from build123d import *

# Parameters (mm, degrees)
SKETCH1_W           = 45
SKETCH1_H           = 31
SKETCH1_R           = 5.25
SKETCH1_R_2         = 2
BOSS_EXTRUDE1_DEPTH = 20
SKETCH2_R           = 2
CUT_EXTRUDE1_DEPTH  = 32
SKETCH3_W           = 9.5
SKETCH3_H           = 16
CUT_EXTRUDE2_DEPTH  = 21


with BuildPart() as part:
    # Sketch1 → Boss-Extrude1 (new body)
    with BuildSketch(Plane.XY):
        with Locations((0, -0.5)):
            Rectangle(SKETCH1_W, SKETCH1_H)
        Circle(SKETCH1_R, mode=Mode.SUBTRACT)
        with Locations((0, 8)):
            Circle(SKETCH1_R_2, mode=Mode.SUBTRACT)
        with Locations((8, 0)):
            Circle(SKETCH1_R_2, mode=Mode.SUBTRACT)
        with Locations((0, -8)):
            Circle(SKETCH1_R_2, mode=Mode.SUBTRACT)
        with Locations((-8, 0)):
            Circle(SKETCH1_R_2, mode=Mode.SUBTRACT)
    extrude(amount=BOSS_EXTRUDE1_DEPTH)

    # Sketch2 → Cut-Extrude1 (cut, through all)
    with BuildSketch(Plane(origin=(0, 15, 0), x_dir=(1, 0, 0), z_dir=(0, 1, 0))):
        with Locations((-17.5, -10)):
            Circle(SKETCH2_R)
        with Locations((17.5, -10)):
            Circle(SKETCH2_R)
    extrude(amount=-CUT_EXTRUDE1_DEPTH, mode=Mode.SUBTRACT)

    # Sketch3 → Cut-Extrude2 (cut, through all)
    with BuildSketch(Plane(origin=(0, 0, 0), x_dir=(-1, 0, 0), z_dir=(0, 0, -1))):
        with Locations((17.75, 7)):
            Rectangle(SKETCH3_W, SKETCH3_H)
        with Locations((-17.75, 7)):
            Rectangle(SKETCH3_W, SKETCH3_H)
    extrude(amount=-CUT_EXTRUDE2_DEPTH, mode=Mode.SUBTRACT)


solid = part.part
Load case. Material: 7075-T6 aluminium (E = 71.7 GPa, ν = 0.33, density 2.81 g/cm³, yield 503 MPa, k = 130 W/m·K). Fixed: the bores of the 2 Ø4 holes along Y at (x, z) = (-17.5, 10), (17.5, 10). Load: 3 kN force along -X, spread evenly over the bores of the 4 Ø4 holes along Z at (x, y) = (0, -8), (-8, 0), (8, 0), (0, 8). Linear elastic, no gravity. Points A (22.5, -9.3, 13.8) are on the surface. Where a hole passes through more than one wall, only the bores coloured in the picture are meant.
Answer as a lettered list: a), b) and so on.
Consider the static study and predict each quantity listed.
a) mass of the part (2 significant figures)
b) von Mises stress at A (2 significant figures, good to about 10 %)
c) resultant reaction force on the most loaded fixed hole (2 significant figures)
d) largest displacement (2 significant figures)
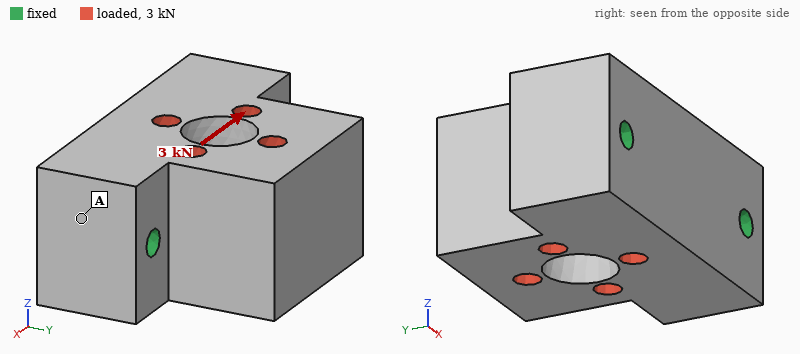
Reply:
a) 53 g
b) 4.1 MPa
c) 1.6 kN
d) 5.9 µm
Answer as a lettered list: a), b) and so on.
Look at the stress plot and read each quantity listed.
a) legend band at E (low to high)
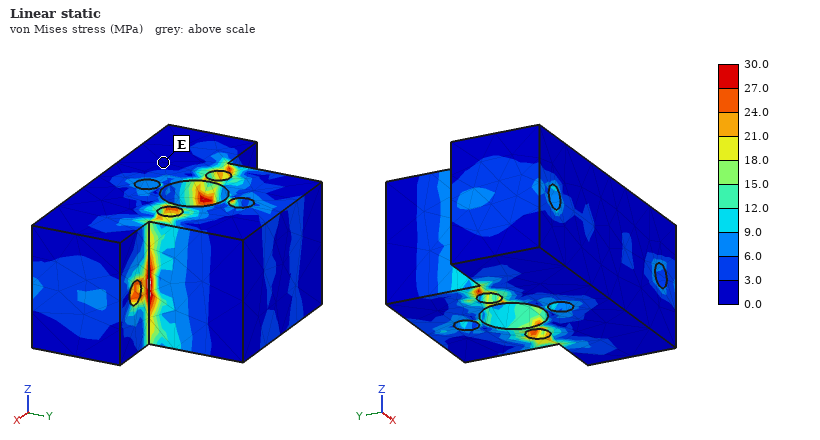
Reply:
a) 0.0 to 3.0 MPa
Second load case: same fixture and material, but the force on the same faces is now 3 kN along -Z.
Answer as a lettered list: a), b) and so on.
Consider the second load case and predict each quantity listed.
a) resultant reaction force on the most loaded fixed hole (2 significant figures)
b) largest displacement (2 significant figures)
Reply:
a) 1.5 kN
b) 17 µm
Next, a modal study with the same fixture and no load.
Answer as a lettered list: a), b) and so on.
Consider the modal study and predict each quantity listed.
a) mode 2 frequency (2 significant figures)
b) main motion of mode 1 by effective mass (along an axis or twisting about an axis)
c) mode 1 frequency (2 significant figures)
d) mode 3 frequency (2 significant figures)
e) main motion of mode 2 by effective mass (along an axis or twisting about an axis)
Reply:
a) 19 kHz
b) along Z
c) 12 kHz
d) 24 kHz
e) along X
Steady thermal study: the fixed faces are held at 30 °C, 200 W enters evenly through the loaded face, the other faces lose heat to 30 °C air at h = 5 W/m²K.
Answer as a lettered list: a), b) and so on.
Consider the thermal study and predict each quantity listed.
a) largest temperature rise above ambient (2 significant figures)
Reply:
a) 61 K
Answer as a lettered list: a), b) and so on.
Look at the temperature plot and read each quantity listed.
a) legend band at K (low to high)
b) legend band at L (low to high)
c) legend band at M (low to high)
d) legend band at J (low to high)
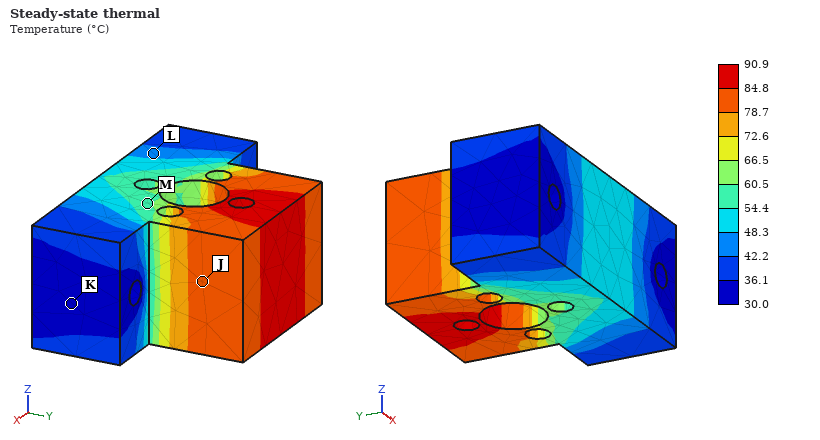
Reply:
a) 30.0 to 36.1 °C
b) 42.2 to 48.3 °C
c) 54.4 to 60.5 °C
d) 78.7 to 84.8 °C
